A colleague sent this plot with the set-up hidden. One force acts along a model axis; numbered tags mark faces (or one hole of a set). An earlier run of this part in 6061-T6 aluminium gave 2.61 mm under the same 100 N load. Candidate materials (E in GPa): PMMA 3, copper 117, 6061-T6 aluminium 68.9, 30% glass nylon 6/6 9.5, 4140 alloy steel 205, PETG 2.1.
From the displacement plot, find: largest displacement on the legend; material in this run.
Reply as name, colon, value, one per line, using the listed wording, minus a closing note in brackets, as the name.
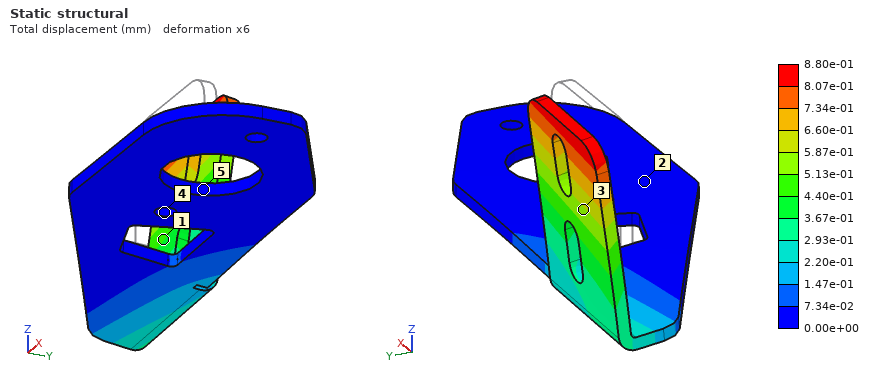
largest displacement on the legend: 8.80e-01 mm
material in this run: 4140 alloy steel
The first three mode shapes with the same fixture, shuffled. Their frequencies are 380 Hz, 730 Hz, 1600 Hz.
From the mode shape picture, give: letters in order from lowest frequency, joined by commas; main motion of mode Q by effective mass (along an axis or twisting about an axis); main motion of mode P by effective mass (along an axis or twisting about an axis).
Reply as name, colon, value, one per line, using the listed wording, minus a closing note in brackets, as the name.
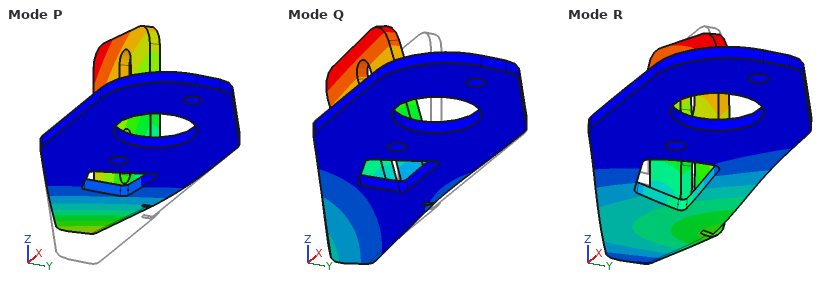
letters in order from lowest frequency, joined by commas: P, Q, R
main motion of mode Q by effective mass: along Y
main motion of mode P by effective mass: along Z
